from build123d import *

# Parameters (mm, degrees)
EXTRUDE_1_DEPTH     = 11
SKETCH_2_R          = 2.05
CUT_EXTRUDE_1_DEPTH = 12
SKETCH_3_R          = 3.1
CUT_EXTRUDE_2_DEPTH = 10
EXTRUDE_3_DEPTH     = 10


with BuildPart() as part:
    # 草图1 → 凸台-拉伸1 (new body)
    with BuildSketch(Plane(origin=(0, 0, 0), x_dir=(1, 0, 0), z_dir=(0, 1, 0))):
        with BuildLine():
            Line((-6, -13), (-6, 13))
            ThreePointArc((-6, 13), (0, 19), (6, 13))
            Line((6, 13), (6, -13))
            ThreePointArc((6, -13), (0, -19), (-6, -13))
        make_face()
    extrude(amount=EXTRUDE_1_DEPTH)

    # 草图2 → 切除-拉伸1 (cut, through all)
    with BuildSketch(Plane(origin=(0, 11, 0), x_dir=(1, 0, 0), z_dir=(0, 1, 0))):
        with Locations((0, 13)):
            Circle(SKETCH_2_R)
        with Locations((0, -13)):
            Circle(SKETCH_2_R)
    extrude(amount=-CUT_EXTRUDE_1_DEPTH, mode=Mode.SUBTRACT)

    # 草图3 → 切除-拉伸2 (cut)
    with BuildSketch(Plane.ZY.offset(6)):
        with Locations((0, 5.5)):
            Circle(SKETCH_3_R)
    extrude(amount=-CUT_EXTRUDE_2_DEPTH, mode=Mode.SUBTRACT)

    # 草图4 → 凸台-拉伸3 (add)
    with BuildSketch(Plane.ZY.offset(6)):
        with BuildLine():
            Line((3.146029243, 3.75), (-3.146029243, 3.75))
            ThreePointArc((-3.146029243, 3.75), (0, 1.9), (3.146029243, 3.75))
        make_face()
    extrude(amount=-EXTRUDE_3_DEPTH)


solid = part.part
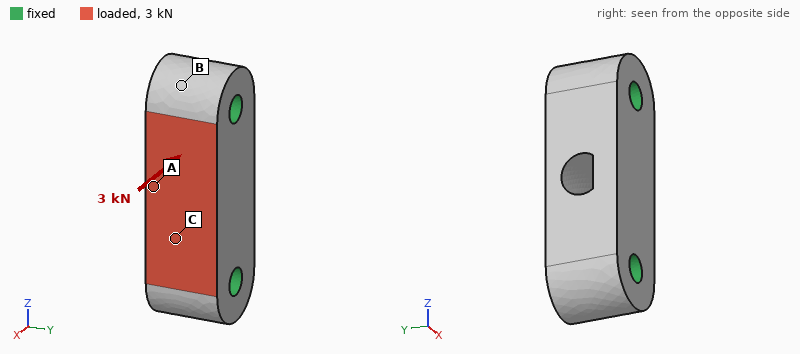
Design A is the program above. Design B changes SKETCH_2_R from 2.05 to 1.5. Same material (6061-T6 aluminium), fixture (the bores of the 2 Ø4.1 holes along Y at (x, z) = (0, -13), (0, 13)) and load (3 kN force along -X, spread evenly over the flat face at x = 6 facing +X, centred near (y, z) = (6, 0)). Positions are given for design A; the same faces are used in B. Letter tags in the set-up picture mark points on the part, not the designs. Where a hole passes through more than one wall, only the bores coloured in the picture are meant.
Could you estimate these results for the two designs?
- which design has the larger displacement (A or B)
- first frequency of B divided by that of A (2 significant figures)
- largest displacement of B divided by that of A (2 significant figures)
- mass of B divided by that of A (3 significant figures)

B
0.87
1.2
1.03
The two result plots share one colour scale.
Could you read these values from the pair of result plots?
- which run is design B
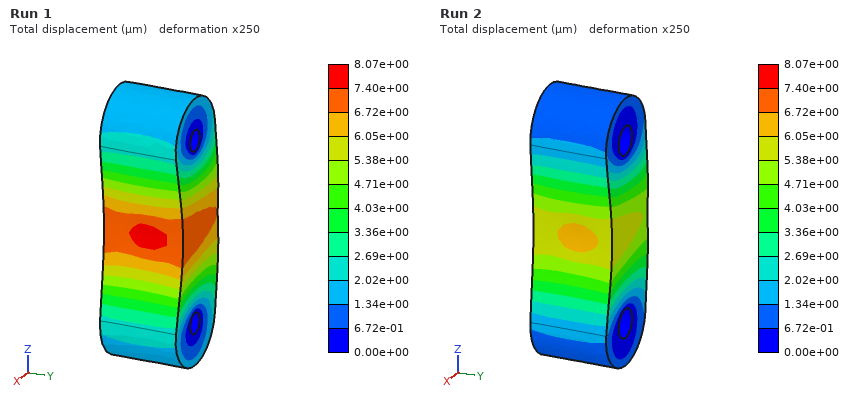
Run 1
